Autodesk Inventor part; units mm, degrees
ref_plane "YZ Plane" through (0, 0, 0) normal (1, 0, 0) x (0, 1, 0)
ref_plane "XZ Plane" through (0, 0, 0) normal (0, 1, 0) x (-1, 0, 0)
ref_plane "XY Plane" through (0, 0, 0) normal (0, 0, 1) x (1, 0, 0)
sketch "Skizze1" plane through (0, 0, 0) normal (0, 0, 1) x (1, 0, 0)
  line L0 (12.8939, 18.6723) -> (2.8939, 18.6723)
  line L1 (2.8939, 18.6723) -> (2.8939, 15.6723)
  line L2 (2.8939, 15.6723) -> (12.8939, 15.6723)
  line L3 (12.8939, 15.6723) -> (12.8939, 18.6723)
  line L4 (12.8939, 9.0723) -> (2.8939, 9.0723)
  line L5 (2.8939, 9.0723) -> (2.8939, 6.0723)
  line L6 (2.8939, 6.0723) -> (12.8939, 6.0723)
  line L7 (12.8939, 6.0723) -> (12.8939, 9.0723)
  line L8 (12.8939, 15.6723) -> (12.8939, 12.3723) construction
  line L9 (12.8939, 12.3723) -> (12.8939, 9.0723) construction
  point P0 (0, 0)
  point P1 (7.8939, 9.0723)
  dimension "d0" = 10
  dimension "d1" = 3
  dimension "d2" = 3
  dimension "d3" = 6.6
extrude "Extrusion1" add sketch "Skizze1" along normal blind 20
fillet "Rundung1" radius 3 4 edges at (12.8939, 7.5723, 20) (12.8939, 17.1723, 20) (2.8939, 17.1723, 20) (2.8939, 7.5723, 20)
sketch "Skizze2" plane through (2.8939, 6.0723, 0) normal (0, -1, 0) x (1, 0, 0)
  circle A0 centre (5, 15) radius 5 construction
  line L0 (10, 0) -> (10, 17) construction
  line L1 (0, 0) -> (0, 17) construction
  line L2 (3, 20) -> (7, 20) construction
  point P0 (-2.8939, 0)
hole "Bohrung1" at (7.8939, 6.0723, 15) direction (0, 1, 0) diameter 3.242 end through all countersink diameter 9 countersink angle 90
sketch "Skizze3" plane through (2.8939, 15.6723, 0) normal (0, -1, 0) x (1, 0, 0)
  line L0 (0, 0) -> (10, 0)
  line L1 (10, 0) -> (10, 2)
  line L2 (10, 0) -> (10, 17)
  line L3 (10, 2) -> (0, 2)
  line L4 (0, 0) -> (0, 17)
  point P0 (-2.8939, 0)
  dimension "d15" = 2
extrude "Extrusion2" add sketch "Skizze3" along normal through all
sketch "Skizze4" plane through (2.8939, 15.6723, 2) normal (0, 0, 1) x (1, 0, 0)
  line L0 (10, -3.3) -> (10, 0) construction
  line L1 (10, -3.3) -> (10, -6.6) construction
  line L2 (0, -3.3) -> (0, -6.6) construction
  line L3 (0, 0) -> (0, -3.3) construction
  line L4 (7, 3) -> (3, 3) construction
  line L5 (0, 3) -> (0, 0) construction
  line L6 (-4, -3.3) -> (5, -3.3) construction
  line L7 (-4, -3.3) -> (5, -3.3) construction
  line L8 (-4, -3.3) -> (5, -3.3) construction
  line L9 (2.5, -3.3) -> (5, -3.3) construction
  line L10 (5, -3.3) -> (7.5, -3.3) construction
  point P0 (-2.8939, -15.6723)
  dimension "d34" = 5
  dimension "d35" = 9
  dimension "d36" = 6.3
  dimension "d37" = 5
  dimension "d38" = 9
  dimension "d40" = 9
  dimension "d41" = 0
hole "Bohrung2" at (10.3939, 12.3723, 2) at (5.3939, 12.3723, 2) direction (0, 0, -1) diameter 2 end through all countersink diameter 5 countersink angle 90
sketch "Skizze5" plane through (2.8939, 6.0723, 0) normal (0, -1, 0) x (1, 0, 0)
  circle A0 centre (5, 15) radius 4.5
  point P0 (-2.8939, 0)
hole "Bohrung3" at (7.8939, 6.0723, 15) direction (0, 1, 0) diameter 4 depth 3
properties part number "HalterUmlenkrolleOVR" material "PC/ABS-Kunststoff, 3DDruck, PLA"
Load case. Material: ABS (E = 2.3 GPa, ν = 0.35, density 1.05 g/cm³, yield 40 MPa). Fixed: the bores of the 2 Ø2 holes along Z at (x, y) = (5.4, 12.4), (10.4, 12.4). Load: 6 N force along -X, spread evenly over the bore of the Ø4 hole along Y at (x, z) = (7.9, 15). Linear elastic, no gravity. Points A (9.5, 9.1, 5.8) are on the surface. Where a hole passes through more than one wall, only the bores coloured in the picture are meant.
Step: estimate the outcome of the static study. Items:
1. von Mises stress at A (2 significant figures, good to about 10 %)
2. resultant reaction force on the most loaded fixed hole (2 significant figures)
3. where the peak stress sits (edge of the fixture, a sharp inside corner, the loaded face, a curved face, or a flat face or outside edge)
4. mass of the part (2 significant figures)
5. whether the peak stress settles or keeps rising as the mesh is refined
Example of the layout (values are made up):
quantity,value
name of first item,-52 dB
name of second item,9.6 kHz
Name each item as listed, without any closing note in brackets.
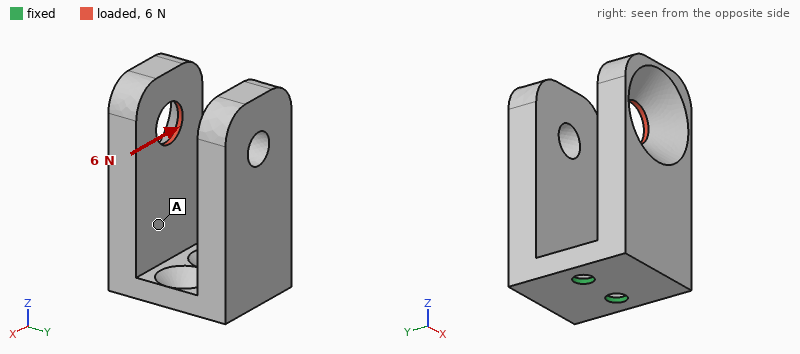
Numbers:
quantity,value
von Mises stress at A,1.9 MPa
resultant reaction force on the most loaded fixed hole,16 N
where the peak stress sits,edge of the fixture
mass of the part,1.2 g
whether the peak stress settles or keeps rising as the mesh is refined,keeps rising
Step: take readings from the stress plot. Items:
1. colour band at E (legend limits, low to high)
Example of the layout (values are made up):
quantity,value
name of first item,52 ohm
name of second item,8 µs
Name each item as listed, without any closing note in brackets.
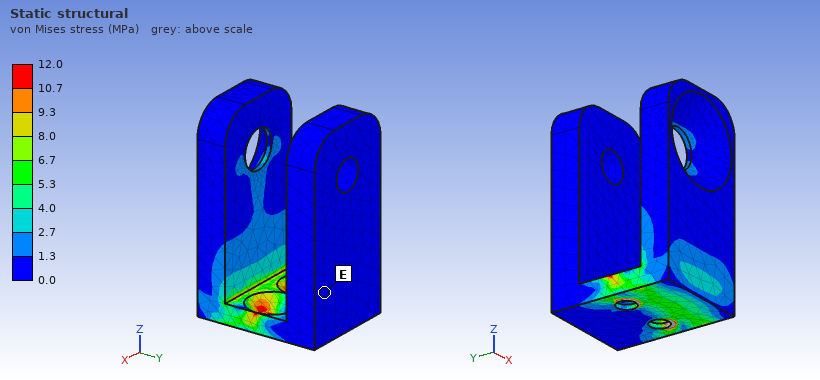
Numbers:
quantity,value
colour band at E,0.0 to 1.3 MPa
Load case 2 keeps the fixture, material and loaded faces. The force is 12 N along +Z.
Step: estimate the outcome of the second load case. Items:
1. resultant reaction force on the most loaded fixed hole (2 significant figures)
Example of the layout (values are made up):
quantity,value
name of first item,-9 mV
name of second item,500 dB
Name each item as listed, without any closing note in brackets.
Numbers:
quantity,value
resultant reaction force on the most loaded fixed hole,6.0 N
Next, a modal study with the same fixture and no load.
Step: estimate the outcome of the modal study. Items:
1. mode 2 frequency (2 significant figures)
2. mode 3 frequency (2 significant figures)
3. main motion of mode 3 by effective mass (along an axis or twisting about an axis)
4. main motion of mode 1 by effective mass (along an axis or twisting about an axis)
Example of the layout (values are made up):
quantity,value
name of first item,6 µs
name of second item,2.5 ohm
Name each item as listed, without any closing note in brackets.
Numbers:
quantity,value
mode 2 frequency,910 Hz
mode 3 frequency,1600 Hz
main motion of mode 3 by effective mass,along X
main motion of mode 1 by effective mass,along Y
